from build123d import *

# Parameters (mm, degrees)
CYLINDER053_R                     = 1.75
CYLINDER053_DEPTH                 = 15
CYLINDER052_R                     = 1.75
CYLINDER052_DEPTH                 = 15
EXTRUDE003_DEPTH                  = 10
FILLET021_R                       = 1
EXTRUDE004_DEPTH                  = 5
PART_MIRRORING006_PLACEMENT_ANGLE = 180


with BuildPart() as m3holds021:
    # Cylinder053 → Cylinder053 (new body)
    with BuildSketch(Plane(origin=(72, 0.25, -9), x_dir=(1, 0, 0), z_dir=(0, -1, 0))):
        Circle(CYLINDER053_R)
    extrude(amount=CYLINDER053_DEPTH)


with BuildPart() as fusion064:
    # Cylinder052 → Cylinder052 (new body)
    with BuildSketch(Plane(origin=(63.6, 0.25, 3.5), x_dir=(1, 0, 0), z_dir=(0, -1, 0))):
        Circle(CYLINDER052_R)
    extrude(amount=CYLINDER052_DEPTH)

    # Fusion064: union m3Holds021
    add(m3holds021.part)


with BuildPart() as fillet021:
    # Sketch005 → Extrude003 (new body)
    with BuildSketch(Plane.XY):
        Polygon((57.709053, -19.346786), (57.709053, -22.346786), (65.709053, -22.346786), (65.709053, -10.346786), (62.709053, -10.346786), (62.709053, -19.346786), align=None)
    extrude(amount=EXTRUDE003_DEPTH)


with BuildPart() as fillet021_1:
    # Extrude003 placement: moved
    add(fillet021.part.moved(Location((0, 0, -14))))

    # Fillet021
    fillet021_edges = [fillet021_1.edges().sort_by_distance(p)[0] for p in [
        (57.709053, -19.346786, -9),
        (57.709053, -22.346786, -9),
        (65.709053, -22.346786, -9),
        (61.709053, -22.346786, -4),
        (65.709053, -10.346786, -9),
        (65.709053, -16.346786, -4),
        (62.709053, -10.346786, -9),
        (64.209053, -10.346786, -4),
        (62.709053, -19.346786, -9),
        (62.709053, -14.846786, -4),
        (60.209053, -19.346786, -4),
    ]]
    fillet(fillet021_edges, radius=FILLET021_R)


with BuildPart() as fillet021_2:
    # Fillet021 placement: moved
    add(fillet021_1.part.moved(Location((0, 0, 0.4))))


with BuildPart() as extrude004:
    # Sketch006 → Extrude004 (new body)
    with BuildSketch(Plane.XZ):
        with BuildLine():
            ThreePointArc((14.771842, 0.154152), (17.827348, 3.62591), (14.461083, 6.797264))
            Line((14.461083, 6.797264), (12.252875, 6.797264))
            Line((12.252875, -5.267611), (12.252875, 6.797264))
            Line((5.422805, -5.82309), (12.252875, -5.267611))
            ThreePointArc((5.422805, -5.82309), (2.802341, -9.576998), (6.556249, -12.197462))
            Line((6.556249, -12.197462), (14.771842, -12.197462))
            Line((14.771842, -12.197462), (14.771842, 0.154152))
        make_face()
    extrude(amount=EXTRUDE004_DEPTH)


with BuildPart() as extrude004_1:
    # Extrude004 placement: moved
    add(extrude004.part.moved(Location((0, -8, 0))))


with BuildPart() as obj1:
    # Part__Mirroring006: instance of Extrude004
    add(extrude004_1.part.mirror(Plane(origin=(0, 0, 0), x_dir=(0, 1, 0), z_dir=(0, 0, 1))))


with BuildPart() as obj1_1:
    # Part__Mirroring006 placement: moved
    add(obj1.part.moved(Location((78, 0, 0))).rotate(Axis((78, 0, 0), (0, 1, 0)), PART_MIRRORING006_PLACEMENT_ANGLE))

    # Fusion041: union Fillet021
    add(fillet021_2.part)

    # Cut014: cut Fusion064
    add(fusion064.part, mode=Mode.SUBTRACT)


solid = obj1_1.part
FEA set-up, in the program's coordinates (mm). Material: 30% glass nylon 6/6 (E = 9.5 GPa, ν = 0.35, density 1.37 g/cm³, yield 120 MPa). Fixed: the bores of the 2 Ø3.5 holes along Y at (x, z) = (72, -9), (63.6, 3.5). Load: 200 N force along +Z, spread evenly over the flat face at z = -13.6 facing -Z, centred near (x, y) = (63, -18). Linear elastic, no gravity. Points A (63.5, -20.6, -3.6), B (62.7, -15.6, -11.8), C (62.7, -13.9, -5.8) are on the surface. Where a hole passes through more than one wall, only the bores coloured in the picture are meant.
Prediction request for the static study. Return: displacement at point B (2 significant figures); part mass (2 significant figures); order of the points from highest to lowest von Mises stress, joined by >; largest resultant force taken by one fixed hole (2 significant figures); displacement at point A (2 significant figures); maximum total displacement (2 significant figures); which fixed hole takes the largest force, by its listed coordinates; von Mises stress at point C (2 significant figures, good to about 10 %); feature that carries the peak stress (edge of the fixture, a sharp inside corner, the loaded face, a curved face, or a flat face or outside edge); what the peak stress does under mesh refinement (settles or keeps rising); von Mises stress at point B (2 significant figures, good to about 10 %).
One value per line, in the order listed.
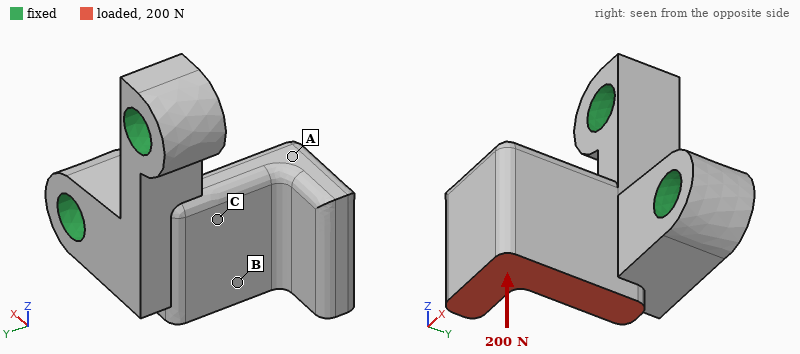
0.070 mm
1.3 g
C > B > A
190 N
0.11 mm
0.16 mm
(63.6, 3.5)
26 MPa
a sharp inside corner
keeps rising
15 MPa
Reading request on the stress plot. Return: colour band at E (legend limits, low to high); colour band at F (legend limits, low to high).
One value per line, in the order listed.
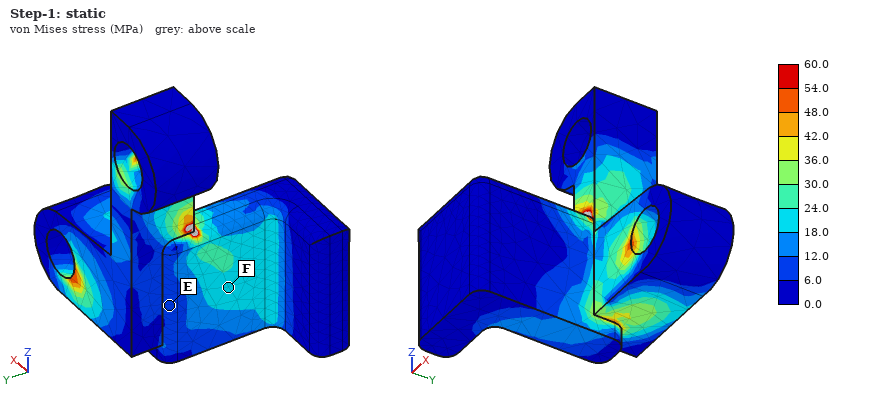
6.0 to 12.0 MPa
18.0 to 24.0 MPa
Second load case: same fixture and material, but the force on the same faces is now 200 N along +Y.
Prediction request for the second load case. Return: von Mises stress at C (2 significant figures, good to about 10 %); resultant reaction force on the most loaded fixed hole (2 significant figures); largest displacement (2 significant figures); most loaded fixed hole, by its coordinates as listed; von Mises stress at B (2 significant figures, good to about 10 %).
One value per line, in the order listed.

18 MPa
210 N
0.32 mm
(72, -9)
29 MPa
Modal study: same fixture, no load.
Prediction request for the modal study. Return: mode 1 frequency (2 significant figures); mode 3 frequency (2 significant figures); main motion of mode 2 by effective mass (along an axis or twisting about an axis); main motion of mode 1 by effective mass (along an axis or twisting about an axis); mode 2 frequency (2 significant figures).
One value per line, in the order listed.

4900 Hz
13 kHz
along Z
along X
8600 Hz
